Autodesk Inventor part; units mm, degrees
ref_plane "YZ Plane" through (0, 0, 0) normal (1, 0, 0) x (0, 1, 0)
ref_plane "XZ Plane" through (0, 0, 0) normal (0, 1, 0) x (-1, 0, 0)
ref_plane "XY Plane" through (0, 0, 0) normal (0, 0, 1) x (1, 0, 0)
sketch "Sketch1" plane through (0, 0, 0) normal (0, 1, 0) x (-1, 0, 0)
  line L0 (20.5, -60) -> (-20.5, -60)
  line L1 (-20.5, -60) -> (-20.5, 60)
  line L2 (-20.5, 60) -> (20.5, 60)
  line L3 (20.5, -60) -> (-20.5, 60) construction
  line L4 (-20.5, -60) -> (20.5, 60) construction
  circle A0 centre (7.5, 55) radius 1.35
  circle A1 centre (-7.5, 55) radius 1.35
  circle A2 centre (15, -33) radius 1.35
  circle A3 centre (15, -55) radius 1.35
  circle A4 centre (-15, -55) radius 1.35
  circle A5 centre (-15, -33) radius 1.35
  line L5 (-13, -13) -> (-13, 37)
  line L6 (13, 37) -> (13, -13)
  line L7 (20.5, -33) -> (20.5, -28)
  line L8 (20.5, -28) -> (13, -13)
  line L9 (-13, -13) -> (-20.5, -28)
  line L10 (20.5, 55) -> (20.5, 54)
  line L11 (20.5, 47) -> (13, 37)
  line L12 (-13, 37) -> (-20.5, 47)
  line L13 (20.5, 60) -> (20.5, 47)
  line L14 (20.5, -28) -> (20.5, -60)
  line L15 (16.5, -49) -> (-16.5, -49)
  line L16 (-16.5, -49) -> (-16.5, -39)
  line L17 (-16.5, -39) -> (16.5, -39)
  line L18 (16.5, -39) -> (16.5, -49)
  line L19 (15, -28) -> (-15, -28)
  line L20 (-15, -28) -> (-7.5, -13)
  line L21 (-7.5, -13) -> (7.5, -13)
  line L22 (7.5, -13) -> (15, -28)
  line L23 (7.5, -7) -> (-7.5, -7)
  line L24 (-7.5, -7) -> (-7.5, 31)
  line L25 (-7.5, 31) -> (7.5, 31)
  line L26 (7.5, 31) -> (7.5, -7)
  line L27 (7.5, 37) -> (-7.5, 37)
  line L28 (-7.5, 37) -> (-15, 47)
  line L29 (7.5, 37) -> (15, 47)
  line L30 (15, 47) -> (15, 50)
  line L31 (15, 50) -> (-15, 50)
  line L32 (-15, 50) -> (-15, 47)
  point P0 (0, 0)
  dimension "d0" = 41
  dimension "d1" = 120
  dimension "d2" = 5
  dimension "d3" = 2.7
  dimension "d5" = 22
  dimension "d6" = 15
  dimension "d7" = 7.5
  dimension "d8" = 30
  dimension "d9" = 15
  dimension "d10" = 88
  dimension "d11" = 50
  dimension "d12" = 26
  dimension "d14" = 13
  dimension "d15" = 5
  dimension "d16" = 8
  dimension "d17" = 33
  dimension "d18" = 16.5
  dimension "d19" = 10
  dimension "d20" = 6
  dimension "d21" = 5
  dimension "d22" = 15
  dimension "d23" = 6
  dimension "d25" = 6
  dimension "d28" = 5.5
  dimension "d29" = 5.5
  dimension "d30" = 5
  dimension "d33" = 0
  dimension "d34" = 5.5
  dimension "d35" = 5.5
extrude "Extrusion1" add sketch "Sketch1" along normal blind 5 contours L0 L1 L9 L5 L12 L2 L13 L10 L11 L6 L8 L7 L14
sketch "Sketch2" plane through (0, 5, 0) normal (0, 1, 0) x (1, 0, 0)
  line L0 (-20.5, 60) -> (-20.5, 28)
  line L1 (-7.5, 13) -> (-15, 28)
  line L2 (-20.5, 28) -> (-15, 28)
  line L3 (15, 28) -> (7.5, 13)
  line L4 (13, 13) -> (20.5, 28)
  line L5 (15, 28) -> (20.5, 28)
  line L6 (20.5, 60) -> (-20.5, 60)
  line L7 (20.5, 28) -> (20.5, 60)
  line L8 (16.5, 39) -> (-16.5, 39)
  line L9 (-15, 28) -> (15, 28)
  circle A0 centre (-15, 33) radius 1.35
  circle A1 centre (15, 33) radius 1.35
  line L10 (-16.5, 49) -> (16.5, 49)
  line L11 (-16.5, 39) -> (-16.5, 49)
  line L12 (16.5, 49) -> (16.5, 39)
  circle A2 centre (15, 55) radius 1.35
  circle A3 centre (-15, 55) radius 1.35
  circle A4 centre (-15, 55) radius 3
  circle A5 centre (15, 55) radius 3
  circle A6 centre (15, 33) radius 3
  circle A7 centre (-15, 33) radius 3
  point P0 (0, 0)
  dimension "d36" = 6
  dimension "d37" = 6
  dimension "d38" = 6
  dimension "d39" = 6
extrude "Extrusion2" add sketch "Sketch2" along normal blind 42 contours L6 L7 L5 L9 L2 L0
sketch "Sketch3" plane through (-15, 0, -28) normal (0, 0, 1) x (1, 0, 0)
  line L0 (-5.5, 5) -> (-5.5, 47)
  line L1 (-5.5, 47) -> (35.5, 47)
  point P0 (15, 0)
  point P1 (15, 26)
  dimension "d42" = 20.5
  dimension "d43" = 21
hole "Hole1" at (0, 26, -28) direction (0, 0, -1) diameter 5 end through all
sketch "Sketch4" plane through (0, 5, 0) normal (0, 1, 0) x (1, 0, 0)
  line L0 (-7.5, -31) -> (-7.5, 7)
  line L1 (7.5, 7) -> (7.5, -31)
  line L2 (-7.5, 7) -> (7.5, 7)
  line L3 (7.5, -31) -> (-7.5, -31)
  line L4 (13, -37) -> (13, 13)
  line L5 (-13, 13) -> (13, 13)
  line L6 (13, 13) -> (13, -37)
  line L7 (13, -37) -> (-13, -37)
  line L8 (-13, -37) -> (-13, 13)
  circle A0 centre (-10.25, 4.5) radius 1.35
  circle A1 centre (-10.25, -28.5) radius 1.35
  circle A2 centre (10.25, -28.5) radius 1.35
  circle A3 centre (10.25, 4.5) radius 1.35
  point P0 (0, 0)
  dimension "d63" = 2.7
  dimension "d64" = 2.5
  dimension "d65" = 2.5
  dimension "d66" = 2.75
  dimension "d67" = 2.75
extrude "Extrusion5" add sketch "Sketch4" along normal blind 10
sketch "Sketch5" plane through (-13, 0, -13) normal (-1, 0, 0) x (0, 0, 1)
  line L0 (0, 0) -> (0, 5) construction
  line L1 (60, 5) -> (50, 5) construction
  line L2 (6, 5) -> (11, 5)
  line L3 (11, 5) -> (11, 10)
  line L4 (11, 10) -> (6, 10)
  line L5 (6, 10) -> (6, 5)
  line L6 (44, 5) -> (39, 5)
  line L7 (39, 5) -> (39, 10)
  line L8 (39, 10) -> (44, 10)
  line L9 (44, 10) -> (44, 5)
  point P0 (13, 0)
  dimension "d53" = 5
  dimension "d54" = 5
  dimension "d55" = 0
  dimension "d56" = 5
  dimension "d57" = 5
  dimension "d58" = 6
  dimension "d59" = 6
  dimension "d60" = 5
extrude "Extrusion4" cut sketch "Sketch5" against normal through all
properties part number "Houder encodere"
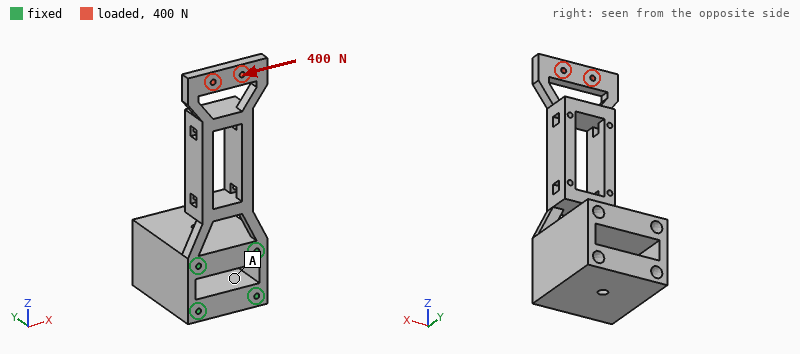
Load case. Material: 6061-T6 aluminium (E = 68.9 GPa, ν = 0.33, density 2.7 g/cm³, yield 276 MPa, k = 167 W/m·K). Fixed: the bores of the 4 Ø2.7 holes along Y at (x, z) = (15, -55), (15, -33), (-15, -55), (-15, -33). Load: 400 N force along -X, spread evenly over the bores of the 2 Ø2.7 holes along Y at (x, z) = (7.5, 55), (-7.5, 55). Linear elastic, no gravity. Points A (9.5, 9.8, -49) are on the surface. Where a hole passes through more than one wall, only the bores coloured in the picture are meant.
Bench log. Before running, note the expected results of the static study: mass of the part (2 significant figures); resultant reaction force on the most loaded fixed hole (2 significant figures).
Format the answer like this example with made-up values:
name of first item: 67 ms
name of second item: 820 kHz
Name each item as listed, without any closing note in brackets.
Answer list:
mass of the part: 150 g
resultant reaction force on the most loaded fixed hole: 1.0 kN
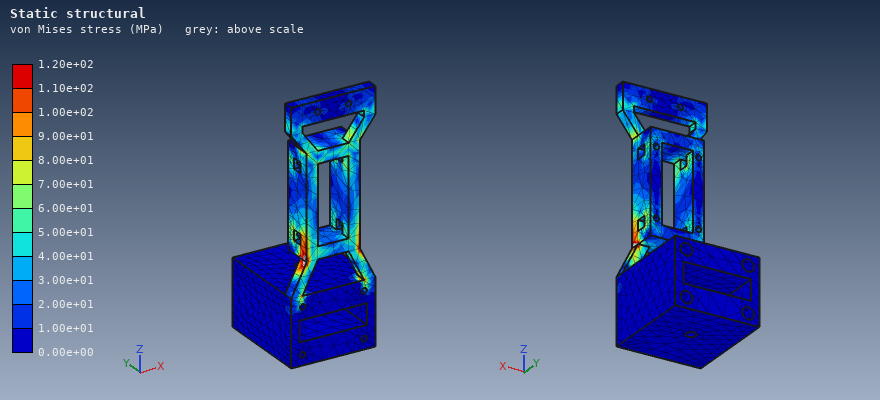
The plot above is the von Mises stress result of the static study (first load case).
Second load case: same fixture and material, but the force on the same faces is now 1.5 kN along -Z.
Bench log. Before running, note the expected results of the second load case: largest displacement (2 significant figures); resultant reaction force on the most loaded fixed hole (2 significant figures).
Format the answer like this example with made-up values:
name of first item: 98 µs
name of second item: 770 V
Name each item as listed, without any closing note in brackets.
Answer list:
largest displacement: 0.14 mm
resultant reaction force on the most loaded fixed hole: 680 N
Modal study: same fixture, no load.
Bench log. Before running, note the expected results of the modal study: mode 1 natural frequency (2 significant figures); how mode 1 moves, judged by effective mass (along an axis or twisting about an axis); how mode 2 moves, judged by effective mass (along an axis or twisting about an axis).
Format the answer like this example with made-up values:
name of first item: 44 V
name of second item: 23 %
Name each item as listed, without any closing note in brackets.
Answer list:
mode 1 natural frequency: 320 Hz
how mode 1 moves, judged by effective mass: along Y
how mode 2 moves, judged by effective mass: along X
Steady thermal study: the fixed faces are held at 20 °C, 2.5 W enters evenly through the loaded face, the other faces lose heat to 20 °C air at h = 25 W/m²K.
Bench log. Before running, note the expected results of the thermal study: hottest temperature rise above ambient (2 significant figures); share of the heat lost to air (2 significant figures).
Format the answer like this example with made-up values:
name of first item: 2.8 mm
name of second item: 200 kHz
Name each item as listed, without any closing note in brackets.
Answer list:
hottest temperature rise above ambient: 13 K
share of the heat lost to air: 50 %
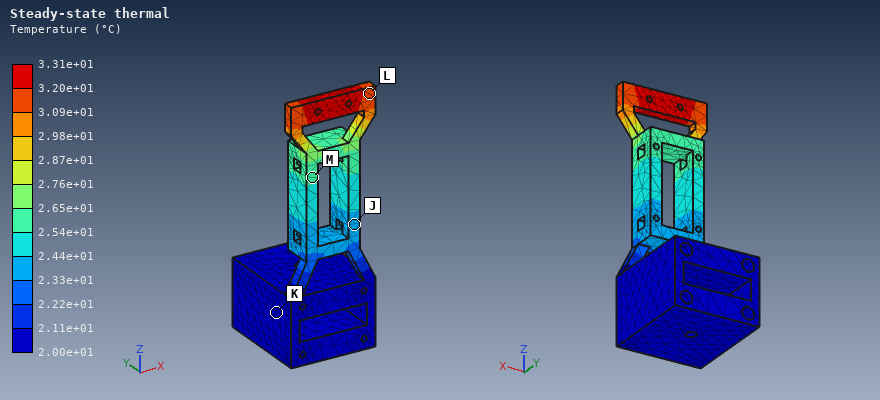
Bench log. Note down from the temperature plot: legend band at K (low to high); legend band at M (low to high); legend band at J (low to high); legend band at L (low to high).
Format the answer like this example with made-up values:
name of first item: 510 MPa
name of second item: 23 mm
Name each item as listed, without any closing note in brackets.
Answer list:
legend band at K: 2.00e+01 to 2.11e+01 °C
legend band at M: 2.54e+01 to 2.65e+01 °C
legend band at J: 2.33e+01 to 2.44e+01 °C
legend band at L: 3.09e+01 to 3.20e+01 °C
